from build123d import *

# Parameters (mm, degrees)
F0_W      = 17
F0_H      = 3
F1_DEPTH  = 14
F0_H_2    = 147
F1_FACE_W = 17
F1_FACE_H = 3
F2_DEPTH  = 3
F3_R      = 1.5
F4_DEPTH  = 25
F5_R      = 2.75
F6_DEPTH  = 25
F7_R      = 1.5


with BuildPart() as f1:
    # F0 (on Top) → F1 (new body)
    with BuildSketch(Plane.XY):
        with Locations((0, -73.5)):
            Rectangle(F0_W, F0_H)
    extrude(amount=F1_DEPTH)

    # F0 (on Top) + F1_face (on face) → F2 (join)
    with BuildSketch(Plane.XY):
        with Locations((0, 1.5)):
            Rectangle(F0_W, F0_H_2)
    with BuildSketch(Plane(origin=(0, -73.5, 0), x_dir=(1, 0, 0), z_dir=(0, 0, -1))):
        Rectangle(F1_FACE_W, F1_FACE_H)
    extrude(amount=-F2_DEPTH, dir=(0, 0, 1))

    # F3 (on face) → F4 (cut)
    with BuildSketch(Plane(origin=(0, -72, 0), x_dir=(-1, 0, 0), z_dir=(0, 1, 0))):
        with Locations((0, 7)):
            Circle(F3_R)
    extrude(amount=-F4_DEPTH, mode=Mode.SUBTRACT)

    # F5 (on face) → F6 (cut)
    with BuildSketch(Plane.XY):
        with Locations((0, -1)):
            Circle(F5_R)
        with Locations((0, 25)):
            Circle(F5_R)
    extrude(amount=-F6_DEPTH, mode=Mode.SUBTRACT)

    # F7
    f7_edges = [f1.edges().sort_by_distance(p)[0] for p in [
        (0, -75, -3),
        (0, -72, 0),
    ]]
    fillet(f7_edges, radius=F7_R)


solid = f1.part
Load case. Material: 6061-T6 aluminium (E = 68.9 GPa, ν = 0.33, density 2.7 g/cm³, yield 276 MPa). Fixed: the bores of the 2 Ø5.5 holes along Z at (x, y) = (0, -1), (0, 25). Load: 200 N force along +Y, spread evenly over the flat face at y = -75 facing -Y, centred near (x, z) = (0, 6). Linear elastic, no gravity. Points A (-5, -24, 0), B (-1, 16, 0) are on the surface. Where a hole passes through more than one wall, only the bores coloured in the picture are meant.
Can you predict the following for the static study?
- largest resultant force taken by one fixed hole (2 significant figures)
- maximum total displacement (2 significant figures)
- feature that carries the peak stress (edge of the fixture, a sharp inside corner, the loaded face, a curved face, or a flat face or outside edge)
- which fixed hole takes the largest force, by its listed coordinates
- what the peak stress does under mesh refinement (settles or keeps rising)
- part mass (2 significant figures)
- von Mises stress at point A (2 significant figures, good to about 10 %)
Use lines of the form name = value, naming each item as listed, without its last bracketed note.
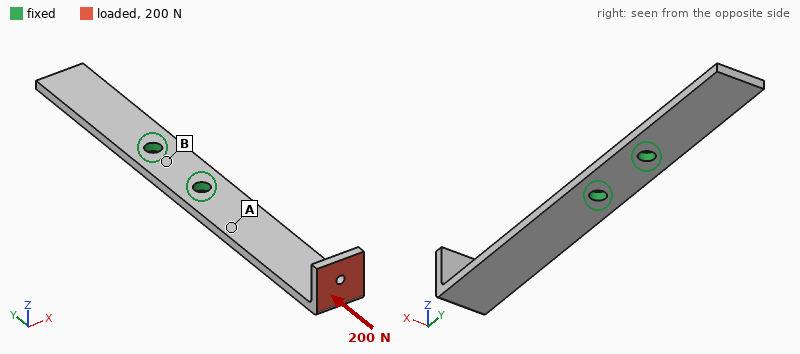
largest resultant force taken by one fixed hole = 190 N
maximum total displacement = 1.7 mm
feature that carries the peak stress = edge of the fixture
which fixed hole takes the largest force, by its listed coordinates = (0, -1)
what the peak stress does under mesh refinement = keeps rising
part mass = 22 g
von Mises stress at point A = 64 MPa
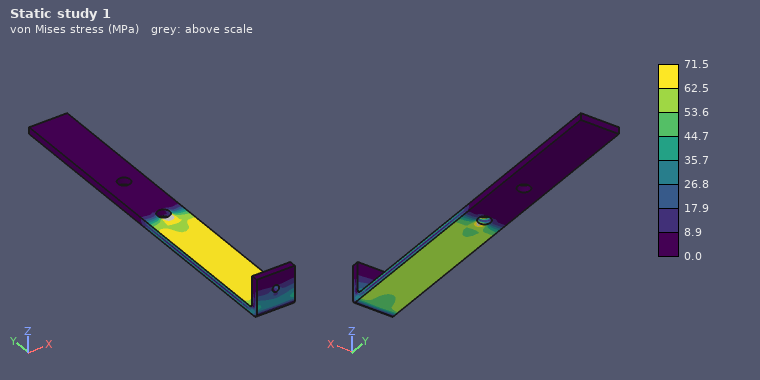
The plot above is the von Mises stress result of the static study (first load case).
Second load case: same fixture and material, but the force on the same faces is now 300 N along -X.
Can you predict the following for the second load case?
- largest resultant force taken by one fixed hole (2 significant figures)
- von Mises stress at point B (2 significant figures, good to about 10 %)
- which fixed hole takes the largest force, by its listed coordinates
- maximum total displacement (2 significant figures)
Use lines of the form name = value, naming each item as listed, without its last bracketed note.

largest resultant force taken by one fixed hole = 710 N
von Mises stress at point B = 21 MPa
which fixed hole takes the largest force, by its listed coordinates = (0, -1)
maximum total displacement = 1.3 mm
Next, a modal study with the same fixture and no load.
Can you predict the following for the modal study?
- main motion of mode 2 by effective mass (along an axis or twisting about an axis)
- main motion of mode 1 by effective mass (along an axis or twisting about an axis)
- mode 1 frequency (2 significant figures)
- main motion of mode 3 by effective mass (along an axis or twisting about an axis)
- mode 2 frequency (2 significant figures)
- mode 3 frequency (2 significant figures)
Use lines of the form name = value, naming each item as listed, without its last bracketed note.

main motion of mode 2 by effective mass = along Z
main motion of mode 1 by effective mass = along Z
mode 1 frequency = 360 Hz
main motion of mode 3 by effective mass = along X
mode 2 frequency = 1100 Hz
mode 3 frequency = 1500 Hz
